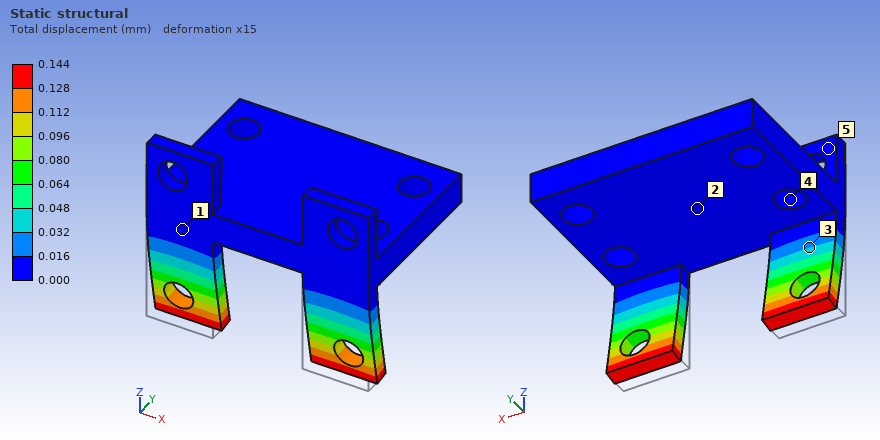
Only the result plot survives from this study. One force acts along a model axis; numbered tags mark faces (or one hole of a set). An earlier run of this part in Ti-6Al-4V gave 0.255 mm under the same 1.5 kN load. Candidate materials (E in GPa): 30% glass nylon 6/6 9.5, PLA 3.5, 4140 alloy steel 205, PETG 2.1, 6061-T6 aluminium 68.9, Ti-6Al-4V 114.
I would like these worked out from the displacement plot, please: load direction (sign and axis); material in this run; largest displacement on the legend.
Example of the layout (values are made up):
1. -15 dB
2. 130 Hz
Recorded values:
1. +Y
2. 4140 alloy steel
3. 0.144 mm
